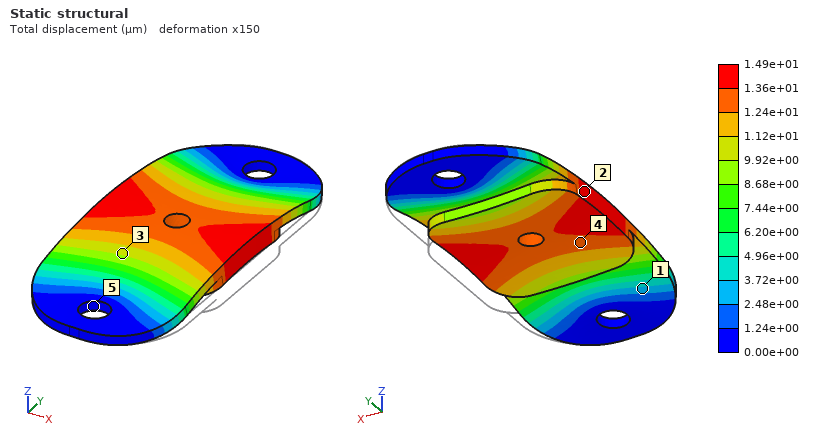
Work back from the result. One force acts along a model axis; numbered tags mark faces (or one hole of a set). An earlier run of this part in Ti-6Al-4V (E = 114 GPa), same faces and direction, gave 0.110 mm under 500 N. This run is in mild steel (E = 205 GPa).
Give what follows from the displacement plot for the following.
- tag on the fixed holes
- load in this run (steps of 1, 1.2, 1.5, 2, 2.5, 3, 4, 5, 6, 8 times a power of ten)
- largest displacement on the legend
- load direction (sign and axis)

5
120 N
1.49e+01 µm
+Z
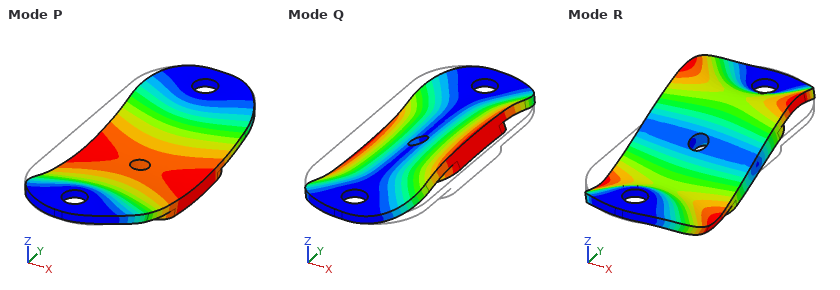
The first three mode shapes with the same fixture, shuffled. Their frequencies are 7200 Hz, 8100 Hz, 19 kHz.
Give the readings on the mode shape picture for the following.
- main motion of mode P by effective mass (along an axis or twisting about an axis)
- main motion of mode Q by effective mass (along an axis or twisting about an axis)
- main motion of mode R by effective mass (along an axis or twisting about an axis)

along Z
twisting about Y
twisting about X
